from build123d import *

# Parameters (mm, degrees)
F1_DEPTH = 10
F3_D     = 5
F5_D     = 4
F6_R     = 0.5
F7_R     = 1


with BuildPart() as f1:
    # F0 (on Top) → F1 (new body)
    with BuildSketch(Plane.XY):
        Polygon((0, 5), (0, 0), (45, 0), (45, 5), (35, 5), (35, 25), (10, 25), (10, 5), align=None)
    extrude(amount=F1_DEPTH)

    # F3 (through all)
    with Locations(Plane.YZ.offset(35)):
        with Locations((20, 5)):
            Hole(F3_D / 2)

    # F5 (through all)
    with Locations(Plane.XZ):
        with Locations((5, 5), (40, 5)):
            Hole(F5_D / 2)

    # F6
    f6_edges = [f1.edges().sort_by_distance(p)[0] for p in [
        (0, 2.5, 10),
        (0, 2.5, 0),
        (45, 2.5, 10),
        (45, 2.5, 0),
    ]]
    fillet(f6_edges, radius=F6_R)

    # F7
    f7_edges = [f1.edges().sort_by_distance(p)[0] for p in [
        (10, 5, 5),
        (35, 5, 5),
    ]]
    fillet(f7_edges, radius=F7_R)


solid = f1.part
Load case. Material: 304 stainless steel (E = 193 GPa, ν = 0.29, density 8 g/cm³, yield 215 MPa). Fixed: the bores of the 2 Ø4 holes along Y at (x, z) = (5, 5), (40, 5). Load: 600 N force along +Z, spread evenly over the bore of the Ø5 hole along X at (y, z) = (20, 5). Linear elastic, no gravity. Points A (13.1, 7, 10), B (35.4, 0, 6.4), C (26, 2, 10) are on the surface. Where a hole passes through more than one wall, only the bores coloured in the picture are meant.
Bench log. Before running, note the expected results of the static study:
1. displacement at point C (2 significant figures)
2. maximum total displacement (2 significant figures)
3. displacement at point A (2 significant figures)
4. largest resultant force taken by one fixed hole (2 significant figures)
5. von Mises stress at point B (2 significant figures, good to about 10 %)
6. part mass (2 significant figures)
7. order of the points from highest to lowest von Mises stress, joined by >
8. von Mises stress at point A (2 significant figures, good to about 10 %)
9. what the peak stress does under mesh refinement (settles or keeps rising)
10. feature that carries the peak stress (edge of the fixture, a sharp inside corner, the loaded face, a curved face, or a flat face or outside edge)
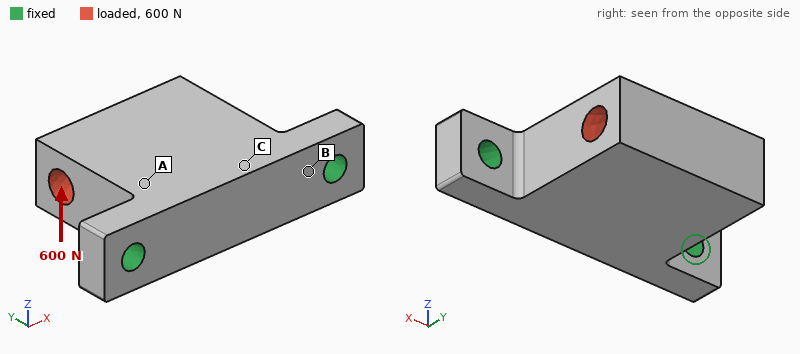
6.2 µm
32 µm
8.7 µm
300 N
65 MPa
53 g
B > A > C
25 MPa
keeps rising
edge of the fixture
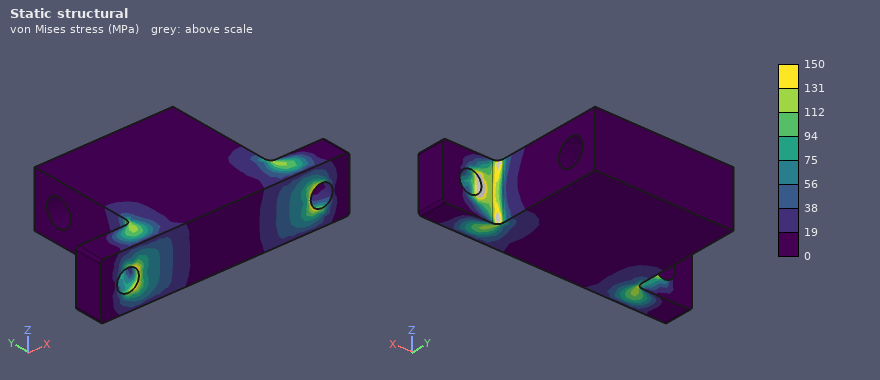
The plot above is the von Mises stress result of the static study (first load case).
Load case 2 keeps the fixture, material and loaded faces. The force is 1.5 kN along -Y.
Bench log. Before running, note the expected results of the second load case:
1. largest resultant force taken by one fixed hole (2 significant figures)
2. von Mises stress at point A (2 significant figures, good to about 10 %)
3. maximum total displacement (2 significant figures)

830 N
15 MPa
3.1 µm
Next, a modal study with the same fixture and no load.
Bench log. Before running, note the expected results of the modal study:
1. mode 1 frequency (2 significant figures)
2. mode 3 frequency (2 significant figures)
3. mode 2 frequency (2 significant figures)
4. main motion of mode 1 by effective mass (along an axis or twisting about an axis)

5300 Hz
18 kHz
17 kHz
along Z
